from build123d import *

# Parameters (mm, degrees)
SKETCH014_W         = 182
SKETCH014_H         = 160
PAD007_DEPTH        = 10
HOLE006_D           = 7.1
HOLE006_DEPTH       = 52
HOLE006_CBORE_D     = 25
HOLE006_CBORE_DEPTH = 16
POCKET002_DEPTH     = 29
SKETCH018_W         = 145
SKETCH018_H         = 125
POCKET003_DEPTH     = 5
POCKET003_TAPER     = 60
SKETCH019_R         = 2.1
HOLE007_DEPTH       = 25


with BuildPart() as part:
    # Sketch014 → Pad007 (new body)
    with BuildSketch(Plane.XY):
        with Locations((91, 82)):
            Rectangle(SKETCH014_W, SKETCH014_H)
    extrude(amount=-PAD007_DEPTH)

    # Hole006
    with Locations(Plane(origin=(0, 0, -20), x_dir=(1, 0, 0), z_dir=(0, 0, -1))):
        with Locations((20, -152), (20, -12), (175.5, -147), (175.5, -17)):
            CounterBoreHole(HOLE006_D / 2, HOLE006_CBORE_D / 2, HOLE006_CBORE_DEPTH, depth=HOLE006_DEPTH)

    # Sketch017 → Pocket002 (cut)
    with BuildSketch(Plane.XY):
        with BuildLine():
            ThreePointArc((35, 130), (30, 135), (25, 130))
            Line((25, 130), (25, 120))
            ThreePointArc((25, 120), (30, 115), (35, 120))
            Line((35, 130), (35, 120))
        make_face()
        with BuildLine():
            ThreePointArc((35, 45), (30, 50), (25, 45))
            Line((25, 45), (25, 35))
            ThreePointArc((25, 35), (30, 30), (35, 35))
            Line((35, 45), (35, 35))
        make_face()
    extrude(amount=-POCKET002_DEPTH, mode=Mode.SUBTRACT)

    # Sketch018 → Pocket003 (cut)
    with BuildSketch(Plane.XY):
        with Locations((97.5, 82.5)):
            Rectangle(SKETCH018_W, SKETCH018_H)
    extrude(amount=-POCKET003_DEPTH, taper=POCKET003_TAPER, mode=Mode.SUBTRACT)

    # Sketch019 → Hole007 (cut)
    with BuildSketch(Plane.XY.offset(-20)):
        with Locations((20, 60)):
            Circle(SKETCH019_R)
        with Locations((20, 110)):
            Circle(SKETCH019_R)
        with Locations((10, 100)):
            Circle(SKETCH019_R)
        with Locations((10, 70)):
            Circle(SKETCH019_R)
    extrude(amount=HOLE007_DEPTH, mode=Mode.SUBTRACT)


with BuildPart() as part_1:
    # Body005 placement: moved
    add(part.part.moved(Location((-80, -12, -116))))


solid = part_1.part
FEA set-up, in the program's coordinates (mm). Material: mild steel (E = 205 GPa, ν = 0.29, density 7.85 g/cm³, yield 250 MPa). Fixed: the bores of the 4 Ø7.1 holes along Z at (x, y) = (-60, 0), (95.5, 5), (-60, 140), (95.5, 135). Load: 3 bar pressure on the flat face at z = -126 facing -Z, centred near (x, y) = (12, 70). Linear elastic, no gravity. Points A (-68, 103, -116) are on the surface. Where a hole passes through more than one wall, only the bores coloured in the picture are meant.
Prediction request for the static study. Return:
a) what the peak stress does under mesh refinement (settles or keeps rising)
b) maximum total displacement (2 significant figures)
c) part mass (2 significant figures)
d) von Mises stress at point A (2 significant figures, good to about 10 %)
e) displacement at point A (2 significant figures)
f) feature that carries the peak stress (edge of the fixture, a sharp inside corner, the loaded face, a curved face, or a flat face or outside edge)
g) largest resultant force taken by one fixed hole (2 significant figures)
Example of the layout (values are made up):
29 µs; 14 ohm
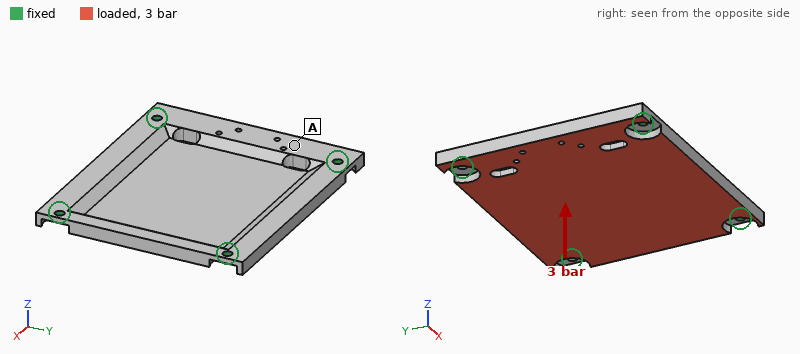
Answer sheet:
keeps rising; 0.20 mm; 1.6 kg; 28 MPa; 0.040 mm; edge of the fixture; 6.5 kN
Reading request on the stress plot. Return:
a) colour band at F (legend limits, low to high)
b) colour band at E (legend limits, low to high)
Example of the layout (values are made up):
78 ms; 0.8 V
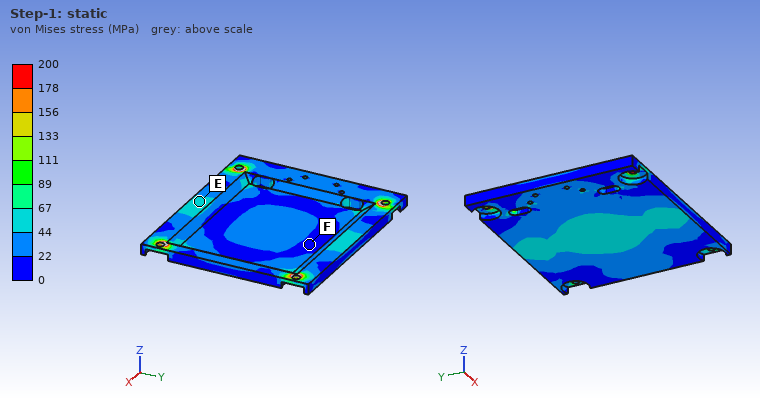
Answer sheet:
0 to 22 MPa; 44 to 67 MPa
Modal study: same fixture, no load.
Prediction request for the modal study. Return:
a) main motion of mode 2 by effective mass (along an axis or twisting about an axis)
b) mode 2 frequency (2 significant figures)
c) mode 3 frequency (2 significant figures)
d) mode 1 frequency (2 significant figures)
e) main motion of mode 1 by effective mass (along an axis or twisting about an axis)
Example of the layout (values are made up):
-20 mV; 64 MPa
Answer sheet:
twisting about X; 1600 Hz; 1800 Hz; 1200 Hz; along Z
